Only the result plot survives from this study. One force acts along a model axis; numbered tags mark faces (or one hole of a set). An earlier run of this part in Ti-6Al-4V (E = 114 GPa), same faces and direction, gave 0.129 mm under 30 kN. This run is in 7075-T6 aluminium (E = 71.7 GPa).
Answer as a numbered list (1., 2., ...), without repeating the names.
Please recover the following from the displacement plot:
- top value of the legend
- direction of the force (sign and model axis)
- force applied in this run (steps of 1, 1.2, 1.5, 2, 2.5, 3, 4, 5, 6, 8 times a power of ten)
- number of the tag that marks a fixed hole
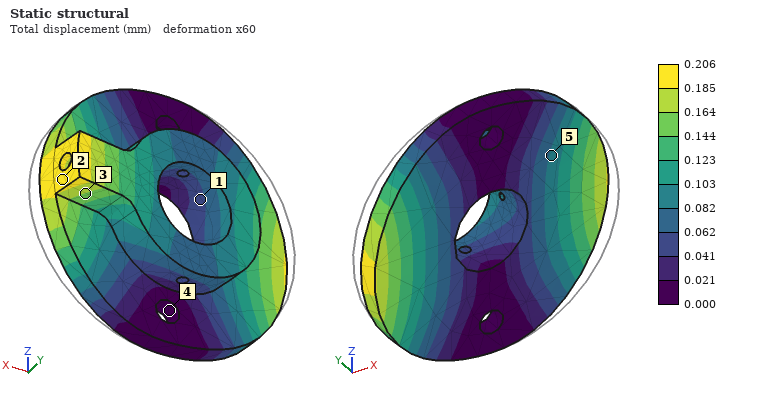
1. 0.206 mm
2. -X
3. 30 kN
4. 4
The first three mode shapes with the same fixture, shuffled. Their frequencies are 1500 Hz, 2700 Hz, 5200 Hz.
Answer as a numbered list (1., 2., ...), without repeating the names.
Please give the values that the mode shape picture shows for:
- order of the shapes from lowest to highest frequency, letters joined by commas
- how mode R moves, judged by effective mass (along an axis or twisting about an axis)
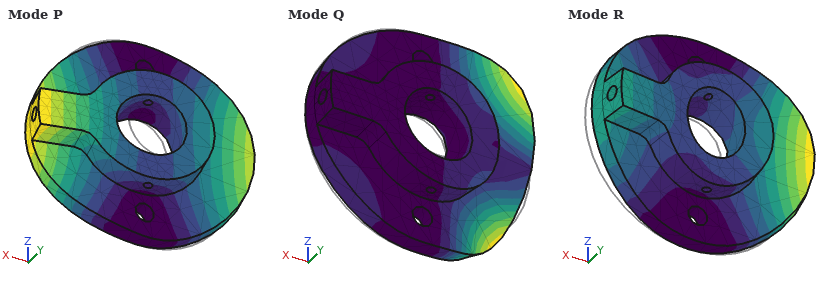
1. P, R, Q
2. along Y
